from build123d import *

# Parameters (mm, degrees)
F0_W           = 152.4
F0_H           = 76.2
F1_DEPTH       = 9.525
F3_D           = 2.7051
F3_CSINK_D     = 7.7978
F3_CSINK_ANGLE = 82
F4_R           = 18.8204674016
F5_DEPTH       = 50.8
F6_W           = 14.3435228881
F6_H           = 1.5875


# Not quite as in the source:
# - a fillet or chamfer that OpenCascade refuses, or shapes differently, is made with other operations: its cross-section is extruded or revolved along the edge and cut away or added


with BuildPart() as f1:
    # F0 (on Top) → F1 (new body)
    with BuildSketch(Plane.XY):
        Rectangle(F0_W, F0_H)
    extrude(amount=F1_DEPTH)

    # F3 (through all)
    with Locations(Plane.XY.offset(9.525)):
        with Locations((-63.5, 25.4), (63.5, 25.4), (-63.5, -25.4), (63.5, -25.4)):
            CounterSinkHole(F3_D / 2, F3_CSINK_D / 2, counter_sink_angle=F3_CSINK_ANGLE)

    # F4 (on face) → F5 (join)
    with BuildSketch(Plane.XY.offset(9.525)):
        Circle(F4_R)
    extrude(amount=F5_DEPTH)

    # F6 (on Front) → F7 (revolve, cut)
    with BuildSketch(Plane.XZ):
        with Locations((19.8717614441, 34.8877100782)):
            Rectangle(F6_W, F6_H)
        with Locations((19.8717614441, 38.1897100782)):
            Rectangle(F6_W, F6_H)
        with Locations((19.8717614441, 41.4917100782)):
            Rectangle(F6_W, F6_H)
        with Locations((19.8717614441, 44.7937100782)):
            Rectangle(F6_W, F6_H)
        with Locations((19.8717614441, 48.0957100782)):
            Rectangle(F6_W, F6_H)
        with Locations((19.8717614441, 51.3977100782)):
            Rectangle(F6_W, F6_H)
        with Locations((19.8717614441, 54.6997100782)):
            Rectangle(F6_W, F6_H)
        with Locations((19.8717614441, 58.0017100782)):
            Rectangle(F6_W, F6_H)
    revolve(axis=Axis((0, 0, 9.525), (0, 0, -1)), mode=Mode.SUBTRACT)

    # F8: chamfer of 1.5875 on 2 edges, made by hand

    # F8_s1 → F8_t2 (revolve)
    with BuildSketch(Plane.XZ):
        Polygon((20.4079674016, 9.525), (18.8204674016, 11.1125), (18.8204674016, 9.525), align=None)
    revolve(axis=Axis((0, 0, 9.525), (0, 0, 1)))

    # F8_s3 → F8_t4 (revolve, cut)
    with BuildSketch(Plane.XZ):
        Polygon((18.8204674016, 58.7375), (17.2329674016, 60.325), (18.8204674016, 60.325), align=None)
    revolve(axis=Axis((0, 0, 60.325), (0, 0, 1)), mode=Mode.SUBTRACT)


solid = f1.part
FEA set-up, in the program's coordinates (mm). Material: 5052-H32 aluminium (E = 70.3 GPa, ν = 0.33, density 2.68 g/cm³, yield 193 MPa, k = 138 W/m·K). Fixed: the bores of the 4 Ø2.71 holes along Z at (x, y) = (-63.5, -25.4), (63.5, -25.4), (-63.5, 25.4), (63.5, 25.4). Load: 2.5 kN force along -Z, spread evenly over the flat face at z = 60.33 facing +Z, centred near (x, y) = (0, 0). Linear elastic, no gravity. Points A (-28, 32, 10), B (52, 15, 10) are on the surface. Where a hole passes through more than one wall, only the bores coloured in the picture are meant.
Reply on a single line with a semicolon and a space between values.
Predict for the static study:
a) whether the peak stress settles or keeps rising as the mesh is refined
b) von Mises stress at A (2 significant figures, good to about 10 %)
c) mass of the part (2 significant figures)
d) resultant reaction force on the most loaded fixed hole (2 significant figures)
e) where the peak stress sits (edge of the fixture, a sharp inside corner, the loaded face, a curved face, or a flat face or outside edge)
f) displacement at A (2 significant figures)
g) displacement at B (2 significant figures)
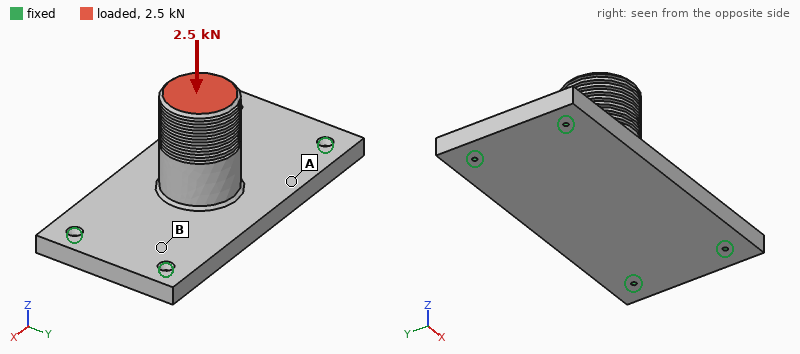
keeps rising; 16 MPa; 430 g; 930 N; edge of the fixture; 61 µm; 23 µm
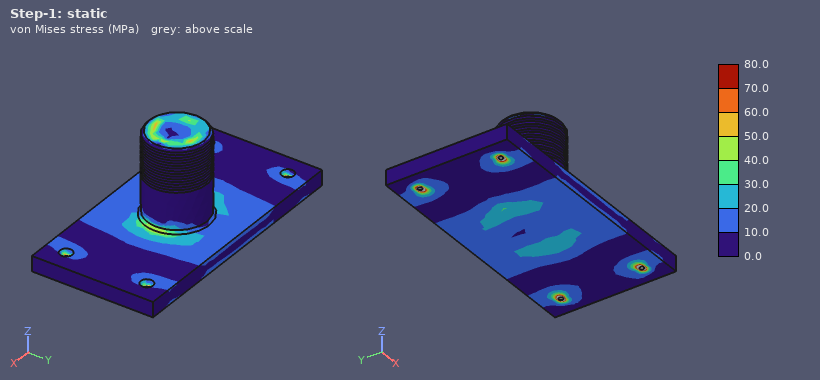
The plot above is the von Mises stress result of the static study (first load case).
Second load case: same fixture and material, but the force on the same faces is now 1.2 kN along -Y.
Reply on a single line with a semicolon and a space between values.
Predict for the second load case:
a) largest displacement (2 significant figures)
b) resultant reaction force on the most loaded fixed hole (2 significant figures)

0.14 mm; 860 N
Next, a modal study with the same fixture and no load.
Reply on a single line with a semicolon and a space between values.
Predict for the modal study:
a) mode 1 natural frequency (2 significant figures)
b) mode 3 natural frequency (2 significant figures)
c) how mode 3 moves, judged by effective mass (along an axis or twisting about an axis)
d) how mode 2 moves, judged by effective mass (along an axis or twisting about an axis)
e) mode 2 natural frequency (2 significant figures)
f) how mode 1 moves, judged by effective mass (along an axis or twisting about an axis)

1700 Hz; 3100 Hz; along X; along Y; 2000 Hz; along Z
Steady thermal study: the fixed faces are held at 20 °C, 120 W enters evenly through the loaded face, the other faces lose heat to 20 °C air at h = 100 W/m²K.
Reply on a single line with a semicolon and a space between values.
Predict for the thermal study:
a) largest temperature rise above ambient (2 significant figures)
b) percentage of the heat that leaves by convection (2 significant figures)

71 K; 66 %
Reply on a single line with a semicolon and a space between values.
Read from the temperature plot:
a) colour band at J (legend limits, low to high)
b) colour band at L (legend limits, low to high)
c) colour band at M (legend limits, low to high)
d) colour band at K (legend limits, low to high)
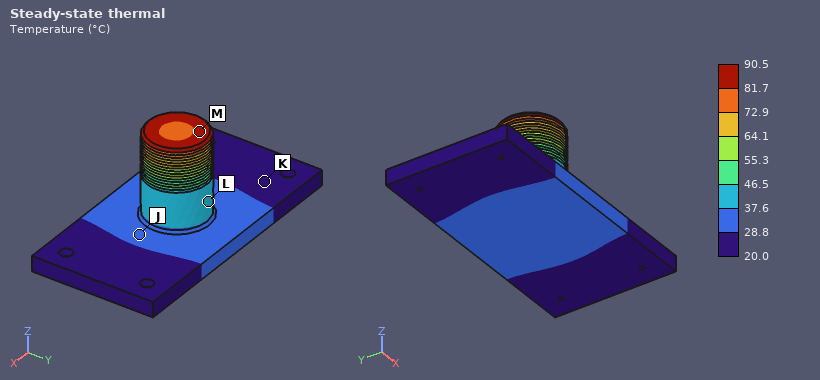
28.8 to 37.6 °C; 37.6 to 46.5 °C; 81.7 to 90.5 °C; 20.0 to 28.8 °C
